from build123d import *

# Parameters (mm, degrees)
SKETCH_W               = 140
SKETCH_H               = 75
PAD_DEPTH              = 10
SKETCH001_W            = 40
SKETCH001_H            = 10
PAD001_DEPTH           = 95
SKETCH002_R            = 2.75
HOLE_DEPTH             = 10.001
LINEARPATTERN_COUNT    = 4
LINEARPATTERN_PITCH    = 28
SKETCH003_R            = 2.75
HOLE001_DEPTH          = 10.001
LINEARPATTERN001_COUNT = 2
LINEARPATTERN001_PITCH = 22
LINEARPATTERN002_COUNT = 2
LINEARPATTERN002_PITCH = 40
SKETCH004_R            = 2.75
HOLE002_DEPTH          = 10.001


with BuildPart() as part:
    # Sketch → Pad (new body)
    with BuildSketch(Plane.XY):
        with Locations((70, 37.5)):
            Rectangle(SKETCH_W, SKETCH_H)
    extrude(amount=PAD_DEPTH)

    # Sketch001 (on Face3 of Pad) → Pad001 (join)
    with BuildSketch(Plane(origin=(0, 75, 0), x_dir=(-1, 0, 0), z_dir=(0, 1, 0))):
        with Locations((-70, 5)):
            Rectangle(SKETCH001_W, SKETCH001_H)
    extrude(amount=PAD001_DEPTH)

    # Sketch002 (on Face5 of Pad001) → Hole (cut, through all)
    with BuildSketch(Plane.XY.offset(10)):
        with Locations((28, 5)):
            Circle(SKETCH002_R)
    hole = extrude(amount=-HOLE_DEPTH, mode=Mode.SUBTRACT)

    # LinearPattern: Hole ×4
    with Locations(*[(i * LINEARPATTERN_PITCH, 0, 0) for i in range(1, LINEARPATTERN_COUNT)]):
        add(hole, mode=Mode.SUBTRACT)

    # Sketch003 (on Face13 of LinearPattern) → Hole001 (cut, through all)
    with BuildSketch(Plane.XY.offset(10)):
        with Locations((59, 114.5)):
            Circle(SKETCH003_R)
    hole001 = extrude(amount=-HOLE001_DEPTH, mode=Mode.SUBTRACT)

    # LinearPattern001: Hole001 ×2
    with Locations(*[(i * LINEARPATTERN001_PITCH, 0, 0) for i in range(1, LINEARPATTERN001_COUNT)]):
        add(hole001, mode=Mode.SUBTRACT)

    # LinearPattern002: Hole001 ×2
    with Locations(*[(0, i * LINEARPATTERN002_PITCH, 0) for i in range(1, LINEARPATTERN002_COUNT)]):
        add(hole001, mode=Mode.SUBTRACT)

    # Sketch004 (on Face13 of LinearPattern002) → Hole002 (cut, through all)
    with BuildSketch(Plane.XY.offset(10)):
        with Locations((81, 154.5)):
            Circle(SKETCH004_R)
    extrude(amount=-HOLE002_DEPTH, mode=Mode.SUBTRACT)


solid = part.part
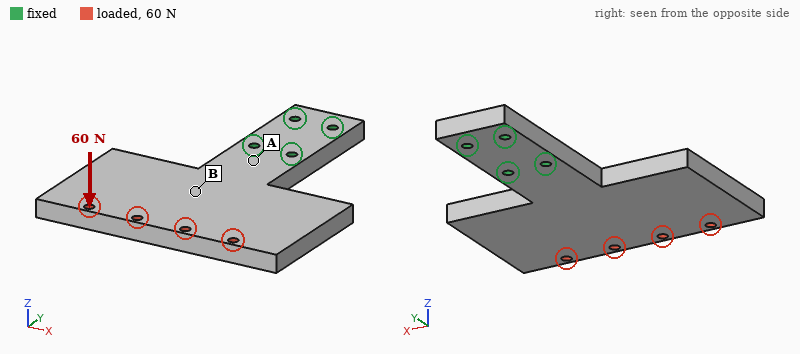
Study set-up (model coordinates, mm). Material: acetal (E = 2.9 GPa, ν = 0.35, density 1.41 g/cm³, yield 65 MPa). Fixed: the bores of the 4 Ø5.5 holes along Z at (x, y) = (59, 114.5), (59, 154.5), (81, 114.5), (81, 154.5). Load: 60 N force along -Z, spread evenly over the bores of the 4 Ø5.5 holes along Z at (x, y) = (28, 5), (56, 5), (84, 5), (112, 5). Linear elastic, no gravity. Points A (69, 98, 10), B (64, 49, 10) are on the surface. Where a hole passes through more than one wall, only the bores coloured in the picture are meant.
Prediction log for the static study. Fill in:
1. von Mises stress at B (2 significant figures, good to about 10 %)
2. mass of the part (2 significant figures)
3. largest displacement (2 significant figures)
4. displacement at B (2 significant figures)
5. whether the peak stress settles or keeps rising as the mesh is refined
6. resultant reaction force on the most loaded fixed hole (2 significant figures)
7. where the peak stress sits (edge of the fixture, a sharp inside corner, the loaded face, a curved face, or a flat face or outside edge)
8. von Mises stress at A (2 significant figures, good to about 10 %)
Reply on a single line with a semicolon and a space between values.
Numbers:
1.8 MPa; 200 g; 2.5 mm; 1.1 mm; keeps rising; 44 N; edge of the fixture; 7.7 MPa
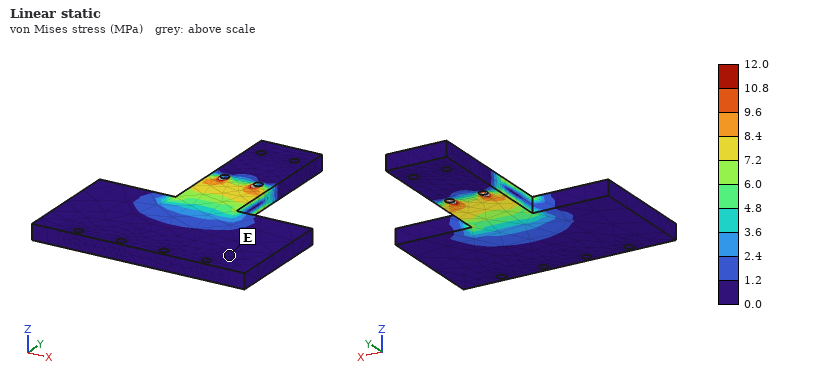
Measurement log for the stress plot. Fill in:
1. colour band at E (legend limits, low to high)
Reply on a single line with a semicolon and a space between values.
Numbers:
0.0 to 1.2 MPa
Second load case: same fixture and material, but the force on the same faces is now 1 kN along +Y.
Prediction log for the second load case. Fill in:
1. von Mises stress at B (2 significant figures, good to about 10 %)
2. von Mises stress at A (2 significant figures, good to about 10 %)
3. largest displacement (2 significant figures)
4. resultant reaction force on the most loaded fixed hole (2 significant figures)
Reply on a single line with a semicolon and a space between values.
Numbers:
1.6 MPa; 2.4 MPa; 84 µm; 470 N
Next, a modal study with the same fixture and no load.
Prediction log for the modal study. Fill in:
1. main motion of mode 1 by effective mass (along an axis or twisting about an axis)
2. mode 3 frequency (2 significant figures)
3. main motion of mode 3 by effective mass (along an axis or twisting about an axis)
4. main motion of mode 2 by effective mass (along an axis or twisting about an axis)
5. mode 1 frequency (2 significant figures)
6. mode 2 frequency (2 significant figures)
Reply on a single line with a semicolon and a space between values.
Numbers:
along Z; 300 Hz; along X; twisting about Y; 100 Hz; 160 Hz
